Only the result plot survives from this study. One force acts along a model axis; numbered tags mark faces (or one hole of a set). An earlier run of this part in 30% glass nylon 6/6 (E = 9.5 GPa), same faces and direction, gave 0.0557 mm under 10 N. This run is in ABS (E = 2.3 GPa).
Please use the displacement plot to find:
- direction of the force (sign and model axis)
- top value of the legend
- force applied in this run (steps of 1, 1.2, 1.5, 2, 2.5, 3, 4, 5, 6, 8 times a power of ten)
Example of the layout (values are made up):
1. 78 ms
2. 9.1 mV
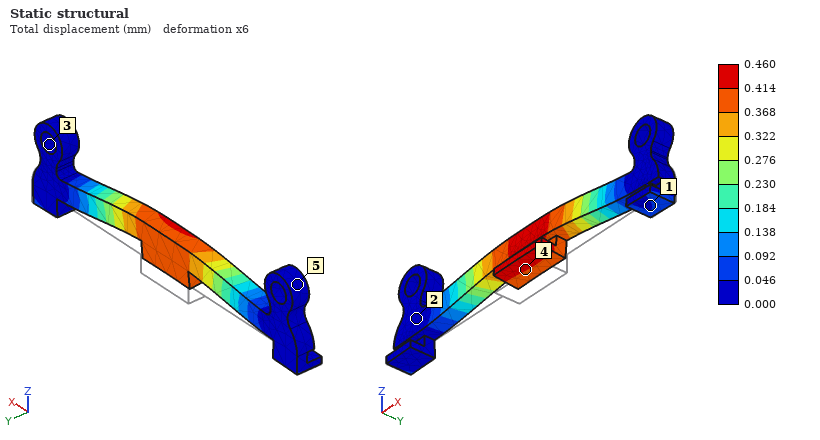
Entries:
1. +Z
2. 0.460 mm
3. 20 N
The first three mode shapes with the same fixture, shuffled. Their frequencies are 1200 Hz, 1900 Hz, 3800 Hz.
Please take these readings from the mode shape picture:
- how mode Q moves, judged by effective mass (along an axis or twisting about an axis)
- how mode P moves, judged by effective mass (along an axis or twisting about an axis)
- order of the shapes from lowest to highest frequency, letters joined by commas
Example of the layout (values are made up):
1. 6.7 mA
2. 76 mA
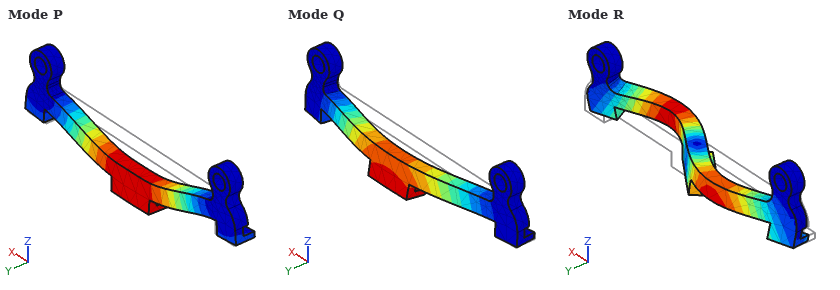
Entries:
1. along Y
2. along Z
3. Q, P, R
